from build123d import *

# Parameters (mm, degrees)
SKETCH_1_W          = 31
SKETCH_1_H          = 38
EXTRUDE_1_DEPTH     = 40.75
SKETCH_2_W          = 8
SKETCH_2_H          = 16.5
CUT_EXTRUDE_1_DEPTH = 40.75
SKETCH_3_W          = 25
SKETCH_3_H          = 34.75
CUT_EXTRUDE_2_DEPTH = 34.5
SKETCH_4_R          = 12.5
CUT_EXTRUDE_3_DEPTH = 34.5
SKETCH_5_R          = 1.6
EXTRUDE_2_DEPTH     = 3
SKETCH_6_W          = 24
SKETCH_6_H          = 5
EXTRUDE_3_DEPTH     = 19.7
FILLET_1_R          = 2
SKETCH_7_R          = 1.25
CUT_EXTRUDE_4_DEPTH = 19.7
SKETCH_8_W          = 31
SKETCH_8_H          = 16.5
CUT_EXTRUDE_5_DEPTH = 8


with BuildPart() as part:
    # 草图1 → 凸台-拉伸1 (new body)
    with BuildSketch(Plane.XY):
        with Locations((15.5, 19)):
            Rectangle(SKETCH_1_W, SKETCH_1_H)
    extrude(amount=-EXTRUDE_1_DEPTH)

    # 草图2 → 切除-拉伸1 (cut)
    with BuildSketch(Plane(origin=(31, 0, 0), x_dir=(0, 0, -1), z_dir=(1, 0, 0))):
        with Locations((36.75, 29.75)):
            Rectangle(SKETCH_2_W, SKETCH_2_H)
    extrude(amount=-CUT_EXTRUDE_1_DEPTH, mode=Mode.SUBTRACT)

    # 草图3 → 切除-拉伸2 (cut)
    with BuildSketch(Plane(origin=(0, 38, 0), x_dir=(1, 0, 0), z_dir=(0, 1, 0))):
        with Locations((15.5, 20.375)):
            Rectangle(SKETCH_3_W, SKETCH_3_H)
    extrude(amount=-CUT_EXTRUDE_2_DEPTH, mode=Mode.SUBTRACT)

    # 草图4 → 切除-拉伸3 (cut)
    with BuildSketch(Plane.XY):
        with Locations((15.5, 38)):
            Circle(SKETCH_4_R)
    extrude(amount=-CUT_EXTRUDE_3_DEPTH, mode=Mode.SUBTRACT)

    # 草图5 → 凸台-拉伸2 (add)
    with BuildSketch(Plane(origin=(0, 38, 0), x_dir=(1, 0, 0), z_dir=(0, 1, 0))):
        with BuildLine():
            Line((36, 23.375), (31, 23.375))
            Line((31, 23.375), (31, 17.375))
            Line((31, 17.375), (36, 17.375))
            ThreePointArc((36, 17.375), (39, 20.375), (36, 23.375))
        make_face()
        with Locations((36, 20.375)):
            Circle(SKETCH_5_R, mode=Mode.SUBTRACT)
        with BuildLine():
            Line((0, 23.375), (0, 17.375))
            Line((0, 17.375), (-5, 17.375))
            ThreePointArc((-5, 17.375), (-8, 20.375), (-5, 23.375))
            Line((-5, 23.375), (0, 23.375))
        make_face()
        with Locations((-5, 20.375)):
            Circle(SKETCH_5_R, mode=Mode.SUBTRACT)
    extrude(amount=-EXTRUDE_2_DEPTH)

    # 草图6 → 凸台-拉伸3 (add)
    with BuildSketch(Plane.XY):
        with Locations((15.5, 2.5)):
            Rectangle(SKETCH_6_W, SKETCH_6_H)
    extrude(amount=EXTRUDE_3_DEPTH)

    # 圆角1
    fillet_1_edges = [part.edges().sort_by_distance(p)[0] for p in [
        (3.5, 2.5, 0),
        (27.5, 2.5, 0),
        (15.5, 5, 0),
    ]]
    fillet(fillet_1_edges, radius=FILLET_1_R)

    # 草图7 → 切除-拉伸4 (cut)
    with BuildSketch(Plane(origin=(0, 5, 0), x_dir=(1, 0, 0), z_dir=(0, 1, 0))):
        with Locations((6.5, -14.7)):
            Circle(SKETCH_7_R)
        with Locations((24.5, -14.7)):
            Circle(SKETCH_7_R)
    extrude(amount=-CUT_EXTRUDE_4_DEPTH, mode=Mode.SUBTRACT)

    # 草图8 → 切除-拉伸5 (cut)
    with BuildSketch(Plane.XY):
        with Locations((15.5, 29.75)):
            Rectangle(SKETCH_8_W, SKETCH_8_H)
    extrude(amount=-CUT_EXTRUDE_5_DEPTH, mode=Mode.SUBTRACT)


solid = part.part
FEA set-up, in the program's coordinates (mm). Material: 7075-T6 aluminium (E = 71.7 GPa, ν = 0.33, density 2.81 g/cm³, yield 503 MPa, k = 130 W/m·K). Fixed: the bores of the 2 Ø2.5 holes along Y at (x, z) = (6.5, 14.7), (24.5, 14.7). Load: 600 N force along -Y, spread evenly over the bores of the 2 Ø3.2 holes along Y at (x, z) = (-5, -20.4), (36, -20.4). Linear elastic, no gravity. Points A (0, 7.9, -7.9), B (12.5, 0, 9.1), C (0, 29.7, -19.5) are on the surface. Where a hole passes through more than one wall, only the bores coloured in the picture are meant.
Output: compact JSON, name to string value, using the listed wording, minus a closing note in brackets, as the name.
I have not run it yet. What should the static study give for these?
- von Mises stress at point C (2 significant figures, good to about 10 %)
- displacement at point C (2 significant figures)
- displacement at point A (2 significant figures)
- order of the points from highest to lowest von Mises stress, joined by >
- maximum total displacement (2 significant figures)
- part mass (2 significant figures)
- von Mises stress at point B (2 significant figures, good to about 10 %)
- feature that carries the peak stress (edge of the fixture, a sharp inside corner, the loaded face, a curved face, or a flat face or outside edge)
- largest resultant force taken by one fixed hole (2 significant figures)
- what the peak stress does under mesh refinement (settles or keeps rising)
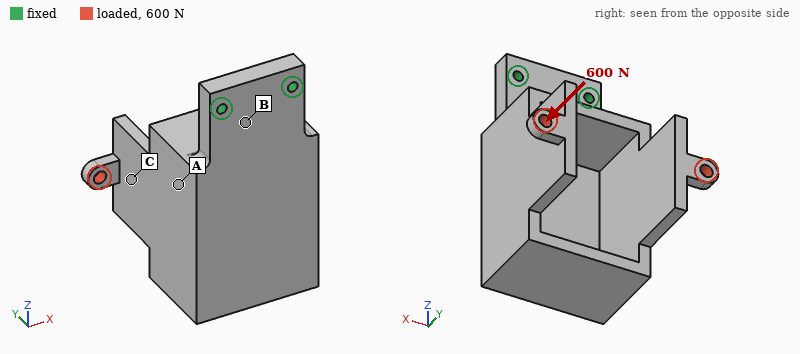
{"von Mises stress at point C": "67 MPa", "displacement at point C": "0.67 mm", "displacement at point A": "0.28 mm", "order of the points from highest to lowest von Mises stress, joined by >": "B > C > A", "maximum total displacement": "0.94 mm", "part mass": "46 g", "von Mises stress at point B": "140 MPa", "feature that carries the peak stress": "edge of the fixture", "largest resultant force taken by one fixed hole": "300 N", "what the peak stress does under mesh refinement": "keeps rising"}
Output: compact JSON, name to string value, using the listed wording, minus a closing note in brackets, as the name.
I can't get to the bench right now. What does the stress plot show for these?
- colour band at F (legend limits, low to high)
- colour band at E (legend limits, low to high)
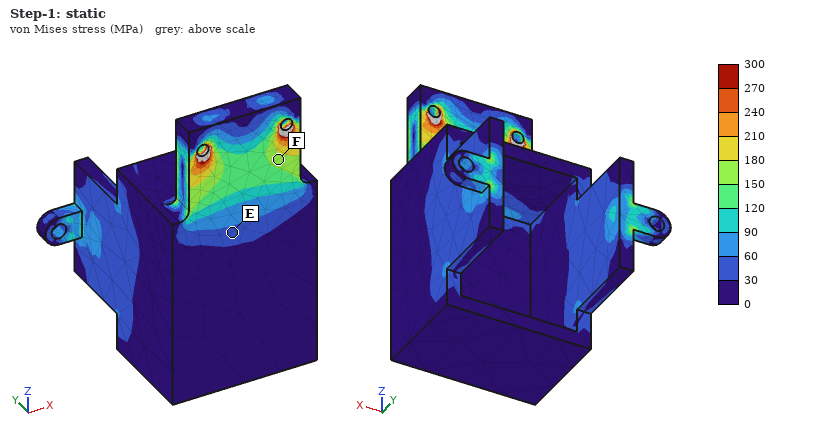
{"colour band at F": "150 to 180 MPa", "colour band at E": "30 to 60 MPa"}
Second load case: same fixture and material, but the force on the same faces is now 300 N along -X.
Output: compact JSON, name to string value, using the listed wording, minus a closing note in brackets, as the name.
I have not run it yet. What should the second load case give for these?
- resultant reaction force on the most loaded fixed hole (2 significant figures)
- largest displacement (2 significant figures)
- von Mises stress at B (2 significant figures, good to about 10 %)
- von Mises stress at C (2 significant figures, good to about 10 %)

{"resultant reaction force on the most loaded fixed hole": "790 N", "largest displacement": "0.49 mm", "von Mises stress at B": "46 MPa", "von Mises stress at C": "41 MPa"}
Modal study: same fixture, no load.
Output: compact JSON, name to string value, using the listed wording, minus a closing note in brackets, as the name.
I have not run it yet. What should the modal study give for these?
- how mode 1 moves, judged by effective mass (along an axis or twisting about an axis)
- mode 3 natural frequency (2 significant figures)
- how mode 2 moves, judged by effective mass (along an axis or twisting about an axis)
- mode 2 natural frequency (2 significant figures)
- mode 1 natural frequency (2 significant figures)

{"how mode 1 moves, judged by effective mass": "along Y", "mode 3 natural frequency": "3300 Hz", "how mode 2 moves, judged by effective mass": "along X", "mode 2 natural frequency": "1500 Hz", "mode 1 natural frequency": "730 Hz"}
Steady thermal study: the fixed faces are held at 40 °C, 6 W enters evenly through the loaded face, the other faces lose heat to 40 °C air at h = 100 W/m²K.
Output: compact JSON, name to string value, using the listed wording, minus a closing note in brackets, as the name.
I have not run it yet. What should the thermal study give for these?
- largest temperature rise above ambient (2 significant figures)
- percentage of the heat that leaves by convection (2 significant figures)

{"largest temperature rise above ambient": "20 K", "percentage of the heat that leaves by convection": "70 %"}
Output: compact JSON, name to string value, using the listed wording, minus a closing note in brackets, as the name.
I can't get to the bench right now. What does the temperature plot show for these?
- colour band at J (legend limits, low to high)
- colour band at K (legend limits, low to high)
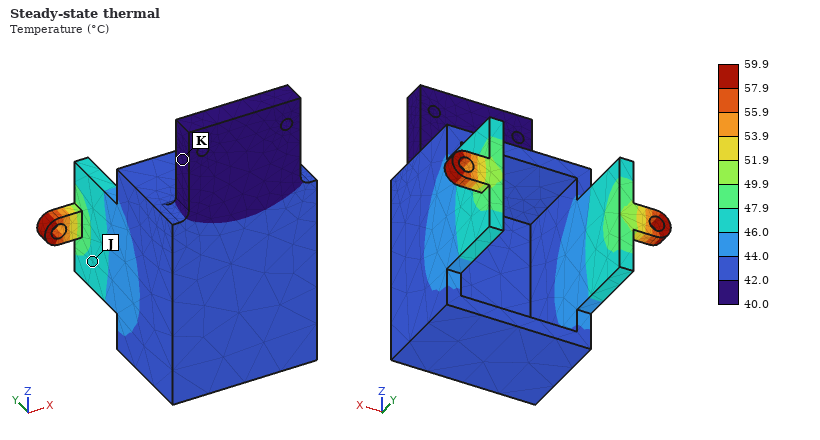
{"colour band at J": "46.0 to 47.9 °C", "colour band at K": "40.0 to 42.0 °C"}
